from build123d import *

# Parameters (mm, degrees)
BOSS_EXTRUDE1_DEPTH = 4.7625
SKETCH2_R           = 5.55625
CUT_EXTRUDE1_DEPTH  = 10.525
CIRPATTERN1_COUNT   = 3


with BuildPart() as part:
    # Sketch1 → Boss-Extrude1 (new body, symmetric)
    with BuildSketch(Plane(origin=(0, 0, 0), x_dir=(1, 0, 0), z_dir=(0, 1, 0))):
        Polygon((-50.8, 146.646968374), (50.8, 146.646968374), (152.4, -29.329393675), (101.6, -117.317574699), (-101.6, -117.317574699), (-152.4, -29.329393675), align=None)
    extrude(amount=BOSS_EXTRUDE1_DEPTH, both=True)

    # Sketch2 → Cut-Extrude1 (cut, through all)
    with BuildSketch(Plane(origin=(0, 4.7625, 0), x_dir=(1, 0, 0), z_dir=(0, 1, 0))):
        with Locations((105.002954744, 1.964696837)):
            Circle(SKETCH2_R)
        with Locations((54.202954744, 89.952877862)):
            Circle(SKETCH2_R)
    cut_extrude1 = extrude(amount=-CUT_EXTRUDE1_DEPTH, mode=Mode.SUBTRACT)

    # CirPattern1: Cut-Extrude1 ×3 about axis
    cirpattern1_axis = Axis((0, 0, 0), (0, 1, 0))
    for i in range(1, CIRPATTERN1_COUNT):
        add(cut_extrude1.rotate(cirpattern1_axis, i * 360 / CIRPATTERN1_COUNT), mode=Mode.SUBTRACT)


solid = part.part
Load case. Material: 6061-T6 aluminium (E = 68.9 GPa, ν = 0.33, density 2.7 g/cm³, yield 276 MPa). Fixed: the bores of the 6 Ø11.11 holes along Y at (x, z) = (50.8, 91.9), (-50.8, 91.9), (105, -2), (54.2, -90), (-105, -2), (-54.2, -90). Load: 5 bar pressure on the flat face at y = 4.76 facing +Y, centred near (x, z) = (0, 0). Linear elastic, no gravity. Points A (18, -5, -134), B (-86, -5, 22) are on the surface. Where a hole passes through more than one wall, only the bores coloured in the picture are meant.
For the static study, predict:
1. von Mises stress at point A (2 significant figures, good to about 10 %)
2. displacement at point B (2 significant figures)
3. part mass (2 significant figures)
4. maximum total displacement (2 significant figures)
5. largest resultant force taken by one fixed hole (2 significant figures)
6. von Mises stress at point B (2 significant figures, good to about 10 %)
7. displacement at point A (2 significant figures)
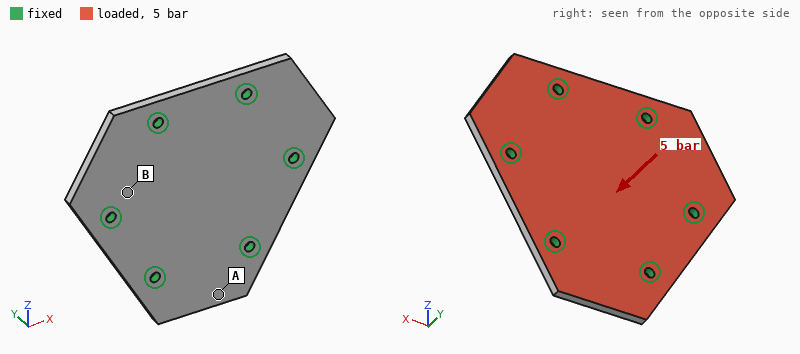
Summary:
14 MPa
0.051 mm
1.5 kg
0.20 mm
4.8 kN
32 MPa
0.11 mm
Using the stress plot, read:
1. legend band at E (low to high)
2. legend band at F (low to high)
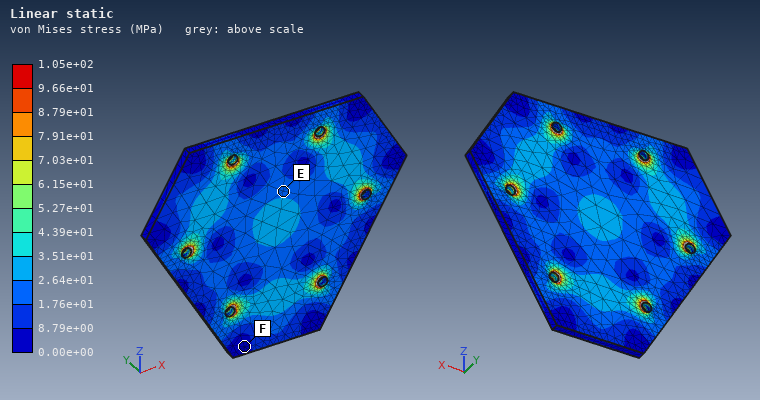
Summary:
1.76e+01 to 2.64e+01 MPa
0.00e+00 to 8.79e+00 MPa
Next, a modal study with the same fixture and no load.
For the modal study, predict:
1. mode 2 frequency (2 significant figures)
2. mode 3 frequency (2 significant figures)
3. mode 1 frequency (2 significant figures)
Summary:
2100 Hz
2100 Hz
1800 Hz
